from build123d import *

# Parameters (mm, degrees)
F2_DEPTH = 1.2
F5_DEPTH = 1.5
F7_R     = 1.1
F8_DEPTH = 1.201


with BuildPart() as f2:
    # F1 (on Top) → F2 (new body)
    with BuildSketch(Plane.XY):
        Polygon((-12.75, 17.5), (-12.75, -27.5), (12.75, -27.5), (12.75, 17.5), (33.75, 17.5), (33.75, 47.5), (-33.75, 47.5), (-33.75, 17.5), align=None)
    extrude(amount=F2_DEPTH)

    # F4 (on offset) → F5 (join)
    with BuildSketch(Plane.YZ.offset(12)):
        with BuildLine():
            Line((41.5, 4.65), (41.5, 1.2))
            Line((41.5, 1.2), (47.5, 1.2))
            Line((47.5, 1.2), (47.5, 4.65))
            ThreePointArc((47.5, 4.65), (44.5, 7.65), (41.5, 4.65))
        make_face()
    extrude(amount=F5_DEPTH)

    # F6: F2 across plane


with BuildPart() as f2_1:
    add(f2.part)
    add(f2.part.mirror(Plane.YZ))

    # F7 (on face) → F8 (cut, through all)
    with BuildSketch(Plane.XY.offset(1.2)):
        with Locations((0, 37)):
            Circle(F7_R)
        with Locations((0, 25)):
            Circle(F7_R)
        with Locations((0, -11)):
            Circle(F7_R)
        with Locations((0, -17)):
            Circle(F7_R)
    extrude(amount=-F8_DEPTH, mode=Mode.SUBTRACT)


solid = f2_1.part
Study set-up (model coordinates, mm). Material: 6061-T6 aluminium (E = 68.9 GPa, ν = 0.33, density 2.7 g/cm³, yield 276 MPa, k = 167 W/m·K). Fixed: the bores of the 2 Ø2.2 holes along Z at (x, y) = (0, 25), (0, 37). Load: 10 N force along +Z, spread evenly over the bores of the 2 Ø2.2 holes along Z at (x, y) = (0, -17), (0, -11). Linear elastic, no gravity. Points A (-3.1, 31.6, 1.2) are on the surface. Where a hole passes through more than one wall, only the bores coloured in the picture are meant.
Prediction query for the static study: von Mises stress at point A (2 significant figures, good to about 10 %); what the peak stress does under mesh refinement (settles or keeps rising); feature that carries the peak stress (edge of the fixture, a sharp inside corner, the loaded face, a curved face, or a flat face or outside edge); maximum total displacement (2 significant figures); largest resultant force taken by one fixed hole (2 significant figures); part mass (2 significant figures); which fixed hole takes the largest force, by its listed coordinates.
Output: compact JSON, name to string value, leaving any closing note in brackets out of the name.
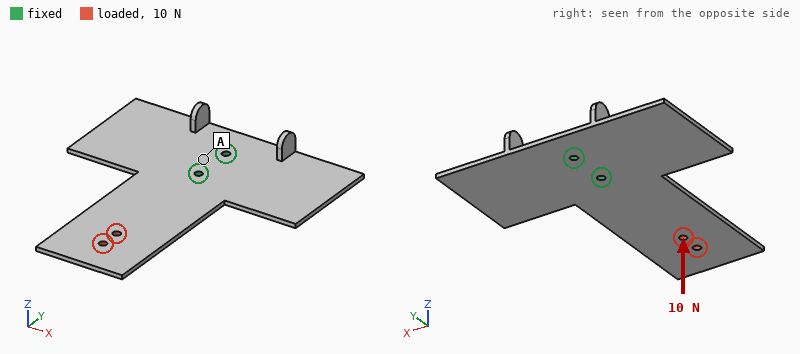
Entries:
{"von Mises stress at point A": "6.6 MPa", "what the peak stress does under mesh refinement": "keeps rising", "feature that carries the peak stress": "edge of the fixture", "maximum total displacement": "1.1 mm", "largest resultant force taken by one fixed hole": "25 N", "part mass": "11 g", "which fixed hole takes the largest force, by its listed coordinates": "(0, 25)"}
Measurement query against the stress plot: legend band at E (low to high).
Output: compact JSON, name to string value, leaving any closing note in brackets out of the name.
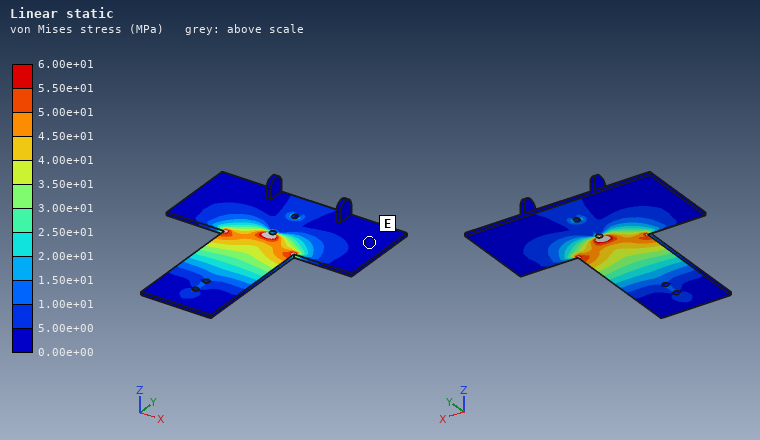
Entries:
{"legend band at E": "0.00e+00 to 5.00e+00 MPa"}
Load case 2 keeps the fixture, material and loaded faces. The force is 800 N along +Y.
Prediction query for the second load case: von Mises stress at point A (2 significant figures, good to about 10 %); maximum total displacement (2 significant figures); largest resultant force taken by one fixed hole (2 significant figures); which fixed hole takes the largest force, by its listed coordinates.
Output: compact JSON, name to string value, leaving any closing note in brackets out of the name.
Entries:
{"von Mises stress at point A": "16 MPa", "maximum total displacement": "22 µm", "largest resultant force taken by one fixed hole": "550 N", "which fixed hole takes the largest force, by its listed coordinates": "(0, 25)"}
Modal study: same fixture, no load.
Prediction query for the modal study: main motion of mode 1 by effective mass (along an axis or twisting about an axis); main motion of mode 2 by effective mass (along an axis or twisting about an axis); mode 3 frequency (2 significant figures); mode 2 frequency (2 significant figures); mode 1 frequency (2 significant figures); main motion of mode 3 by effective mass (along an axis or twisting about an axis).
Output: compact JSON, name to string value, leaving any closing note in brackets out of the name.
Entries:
{"main motion of mode 1 by effective mass": "along Z", "main motion of mode 2 by effective mass": "twisting about Y", "mode 3 frequency": "970 Hz", "mode 2 frequency": "840 Hz", "mode 1 frequency": "370 Hz", "main motion of mode 3 by effective mass": "along Z"}
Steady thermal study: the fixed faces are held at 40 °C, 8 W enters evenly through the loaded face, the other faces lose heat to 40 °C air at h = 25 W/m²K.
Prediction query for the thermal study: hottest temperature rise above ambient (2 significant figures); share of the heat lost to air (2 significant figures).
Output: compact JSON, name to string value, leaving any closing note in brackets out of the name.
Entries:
{"hottest temperature rise above ambient": "55 K", "share of the heat lost to air": "33 %"}
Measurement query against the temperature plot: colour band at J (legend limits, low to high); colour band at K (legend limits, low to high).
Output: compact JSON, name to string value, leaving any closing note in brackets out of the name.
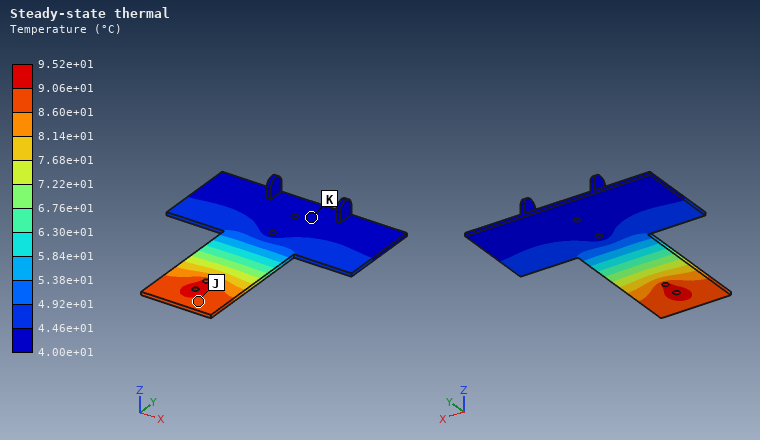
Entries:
{"colour band at J": "8.60e+01 to 9.06e+01 °C", "colour band at K": "4.00e+01 to 4.46e+01 °C"}
